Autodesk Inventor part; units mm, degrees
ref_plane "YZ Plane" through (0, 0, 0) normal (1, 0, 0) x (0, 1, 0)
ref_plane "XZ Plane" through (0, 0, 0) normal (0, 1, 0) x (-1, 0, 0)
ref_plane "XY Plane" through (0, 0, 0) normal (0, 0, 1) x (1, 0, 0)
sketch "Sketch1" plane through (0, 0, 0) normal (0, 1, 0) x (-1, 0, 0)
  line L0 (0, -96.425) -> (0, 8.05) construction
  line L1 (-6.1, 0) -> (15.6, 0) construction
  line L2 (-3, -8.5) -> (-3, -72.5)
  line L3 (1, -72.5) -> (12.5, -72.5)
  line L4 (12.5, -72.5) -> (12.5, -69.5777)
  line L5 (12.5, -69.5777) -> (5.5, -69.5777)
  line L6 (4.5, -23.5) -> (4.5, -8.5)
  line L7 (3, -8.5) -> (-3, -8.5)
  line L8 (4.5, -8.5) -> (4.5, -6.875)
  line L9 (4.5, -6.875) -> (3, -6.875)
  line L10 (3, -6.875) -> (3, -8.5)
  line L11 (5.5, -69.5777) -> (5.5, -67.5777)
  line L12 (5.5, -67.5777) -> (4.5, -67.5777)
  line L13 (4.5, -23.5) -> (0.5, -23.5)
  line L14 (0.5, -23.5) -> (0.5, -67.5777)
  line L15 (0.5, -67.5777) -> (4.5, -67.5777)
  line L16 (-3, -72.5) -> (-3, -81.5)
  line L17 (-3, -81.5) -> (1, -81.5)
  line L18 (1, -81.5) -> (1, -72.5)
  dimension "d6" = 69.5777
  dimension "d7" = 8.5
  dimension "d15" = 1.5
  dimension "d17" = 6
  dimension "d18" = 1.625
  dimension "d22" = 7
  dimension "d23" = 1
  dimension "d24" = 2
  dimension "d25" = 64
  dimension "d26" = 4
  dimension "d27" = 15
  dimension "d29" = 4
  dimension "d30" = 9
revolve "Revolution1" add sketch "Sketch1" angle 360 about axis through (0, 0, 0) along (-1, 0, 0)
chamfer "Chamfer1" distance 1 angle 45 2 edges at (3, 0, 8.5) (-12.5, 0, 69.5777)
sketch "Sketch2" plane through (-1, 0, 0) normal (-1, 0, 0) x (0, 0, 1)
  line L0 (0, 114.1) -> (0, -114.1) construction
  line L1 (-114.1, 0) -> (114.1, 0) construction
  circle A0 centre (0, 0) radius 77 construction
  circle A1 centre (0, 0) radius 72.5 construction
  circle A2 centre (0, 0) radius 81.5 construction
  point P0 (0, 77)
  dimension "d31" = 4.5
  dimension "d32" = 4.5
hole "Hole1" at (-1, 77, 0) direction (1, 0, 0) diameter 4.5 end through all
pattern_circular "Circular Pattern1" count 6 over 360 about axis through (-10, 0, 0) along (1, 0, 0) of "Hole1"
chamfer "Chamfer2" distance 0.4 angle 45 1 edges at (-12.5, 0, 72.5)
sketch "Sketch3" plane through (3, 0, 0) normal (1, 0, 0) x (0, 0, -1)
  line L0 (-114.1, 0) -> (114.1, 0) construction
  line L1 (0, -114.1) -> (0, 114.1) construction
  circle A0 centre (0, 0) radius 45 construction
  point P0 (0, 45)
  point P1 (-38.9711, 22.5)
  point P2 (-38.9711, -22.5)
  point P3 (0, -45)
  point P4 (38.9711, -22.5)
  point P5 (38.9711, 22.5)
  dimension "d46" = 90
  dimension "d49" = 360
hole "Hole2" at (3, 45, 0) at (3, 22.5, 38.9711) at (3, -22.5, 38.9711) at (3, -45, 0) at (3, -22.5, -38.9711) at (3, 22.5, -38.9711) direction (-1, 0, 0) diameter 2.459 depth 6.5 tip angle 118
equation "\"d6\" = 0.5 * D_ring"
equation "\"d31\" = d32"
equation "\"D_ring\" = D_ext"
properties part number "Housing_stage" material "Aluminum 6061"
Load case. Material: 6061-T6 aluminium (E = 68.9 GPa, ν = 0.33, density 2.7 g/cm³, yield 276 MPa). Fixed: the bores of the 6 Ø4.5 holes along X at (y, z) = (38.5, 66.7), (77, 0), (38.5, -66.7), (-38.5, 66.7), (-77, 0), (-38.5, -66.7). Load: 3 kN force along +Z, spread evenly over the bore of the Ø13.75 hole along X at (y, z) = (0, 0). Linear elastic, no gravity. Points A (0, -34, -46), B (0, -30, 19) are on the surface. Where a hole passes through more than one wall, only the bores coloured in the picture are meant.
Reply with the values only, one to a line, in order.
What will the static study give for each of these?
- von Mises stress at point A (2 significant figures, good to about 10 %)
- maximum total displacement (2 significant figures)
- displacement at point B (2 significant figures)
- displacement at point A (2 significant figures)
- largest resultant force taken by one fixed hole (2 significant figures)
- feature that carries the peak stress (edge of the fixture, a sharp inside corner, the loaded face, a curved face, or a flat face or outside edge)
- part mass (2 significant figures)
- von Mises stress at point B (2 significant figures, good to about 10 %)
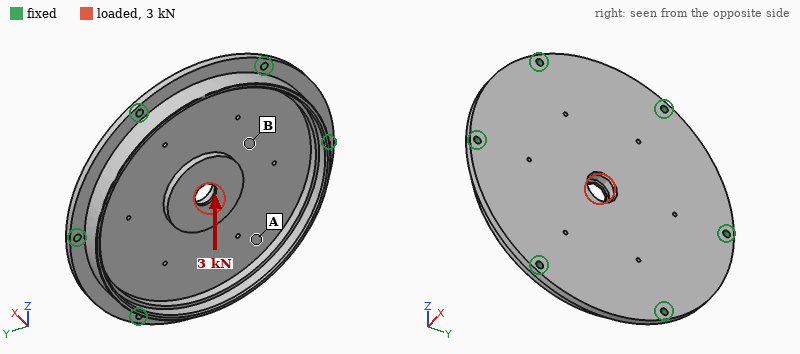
6.9 MPa
45 µm
24 µm
12 µm
680 N
the loaded face
270 g
14 MPa
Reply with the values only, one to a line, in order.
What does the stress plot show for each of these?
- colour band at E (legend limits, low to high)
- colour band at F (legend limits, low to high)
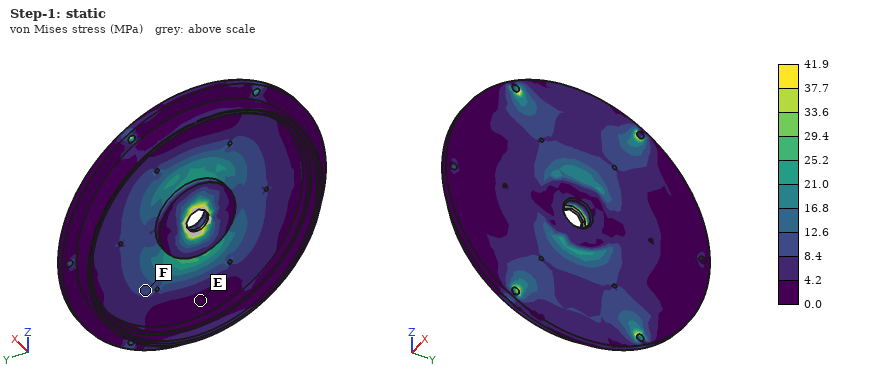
0.0 to 4.2 MPa
8.4 to 12.6 MPa
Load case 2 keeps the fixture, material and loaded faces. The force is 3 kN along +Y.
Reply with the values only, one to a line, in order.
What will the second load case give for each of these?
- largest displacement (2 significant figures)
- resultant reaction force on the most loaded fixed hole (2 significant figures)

45 µm
770 N
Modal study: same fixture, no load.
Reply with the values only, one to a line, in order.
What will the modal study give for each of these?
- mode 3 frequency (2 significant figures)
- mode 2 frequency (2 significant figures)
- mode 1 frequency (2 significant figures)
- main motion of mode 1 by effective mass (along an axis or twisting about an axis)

3000 Hz
3000 Hz
1500 Hz
along X
